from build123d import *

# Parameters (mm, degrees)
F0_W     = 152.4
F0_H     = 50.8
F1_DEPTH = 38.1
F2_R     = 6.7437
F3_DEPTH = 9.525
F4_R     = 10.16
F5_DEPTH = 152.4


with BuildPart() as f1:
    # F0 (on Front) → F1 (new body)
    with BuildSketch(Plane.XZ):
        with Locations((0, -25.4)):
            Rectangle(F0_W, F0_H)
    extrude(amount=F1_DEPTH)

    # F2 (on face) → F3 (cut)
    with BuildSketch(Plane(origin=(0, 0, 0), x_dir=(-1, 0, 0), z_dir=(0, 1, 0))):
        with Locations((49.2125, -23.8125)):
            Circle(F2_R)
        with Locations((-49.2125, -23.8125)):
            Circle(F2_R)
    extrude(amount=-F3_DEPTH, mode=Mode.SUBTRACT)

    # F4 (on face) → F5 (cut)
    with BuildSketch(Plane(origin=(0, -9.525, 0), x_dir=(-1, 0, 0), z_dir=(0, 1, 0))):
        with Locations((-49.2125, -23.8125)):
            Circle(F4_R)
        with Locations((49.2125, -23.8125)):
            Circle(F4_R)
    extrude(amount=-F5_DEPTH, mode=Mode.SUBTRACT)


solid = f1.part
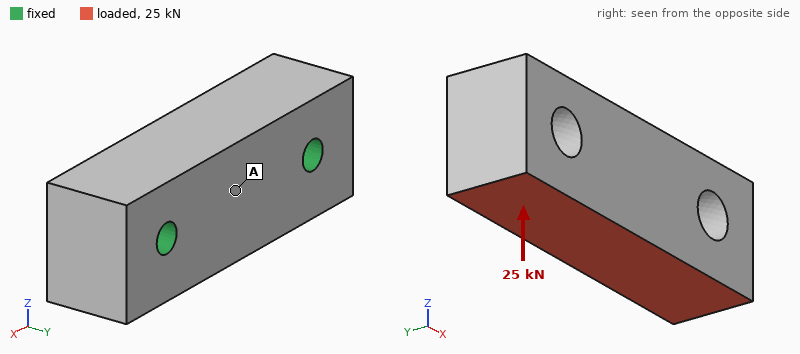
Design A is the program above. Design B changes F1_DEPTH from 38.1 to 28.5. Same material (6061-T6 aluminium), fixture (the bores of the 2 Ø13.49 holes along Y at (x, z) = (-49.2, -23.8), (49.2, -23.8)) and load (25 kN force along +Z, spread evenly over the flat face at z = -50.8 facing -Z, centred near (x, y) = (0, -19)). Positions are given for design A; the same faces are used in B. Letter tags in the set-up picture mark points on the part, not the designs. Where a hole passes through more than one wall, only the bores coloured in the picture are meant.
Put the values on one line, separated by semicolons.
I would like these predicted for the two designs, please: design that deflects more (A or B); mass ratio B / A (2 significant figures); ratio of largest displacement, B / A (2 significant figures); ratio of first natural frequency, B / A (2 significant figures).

A; 0.75; 0.64; 1.4
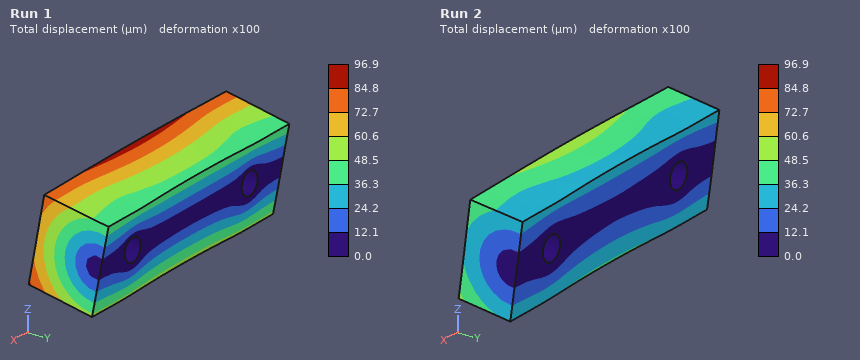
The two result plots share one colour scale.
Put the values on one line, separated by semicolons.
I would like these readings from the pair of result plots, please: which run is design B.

Run 2
